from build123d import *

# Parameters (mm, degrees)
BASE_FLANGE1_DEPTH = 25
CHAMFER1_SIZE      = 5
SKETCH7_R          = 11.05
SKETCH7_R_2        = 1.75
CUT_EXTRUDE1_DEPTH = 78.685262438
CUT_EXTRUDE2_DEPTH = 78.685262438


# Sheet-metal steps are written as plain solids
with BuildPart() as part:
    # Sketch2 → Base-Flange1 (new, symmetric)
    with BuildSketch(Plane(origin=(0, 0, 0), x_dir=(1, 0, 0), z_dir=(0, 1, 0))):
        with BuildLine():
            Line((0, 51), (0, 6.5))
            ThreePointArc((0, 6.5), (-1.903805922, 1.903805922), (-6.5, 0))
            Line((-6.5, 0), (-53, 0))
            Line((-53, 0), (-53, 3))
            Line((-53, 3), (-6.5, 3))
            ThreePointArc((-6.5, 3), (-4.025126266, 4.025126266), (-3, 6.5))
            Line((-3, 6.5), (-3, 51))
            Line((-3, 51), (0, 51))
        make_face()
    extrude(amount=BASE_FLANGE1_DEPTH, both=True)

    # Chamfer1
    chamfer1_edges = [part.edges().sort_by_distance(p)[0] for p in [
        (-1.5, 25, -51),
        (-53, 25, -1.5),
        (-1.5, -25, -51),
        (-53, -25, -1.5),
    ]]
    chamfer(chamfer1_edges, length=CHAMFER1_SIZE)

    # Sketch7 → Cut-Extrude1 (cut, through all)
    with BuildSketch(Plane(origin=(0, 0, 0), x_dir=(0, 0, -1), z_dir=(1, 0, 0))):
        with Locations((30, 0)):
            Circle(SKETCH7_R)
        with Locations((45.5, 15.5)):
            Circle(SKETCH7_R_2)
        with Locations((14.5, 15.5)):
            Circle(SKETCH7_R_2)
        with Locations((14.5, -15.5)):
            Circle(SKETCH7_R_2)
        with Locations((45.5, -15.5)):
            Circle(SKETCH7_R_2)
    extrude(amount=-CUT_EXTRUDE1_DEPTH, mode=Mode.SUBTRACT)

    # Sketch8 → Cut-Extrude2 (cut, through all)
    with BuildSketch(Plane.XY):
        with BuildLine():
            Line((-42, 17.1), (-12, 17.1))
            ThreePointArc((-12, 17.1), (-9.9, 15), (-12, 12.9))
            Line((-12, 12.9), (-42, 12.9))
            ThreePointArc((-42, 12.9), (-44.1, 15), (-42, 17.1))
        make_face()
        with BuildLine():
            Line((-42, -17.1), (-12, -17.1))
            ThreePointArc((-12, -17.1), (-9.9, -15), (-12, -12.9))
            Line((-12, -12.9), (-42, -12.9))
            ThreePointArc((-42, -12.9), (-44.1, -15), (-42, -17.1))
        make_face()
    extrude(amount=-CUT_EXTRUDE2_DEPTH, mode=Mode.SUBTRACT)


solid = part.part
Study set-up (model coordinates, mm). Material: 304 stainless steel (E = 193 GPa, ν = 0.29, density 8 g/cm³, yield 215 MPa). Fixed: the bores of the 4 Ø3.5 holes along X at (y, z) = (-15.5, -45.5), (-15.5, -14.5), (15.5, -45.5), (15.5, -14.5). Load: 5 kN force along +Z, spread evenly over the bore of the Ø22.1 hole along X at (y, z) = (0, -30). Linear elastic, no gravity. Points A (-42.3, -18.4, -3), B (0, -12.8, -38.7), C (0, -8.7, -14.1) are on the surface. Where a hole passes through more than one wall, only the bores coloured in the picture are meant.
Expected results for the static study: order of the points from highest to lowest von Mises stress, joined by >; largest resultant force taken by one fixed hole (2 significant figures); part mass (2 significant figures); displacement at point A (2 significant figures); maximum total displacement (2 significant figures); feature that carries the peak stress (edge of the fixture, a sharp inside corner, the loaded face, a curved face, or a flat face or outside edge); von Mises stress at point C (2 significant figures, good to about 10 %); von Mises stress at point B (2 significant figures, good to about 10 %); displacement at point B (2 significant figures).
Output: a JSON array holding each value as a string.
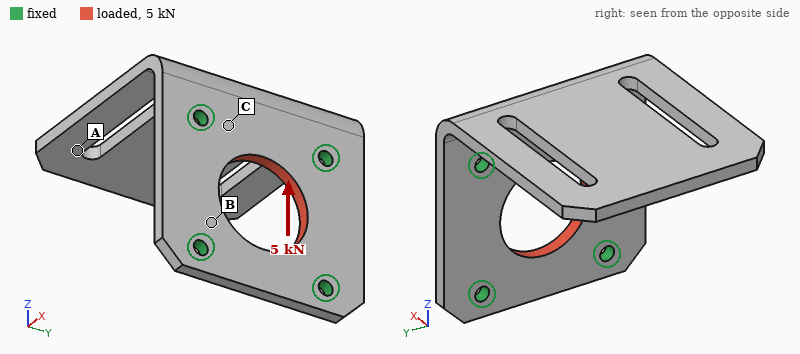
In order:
["B > C > A", "1.3 kN", "100 g", "1.8 µm", "5.4 µm", "edge of the fixture", "20 MPa", "36 MPa", "1.6 µm"]
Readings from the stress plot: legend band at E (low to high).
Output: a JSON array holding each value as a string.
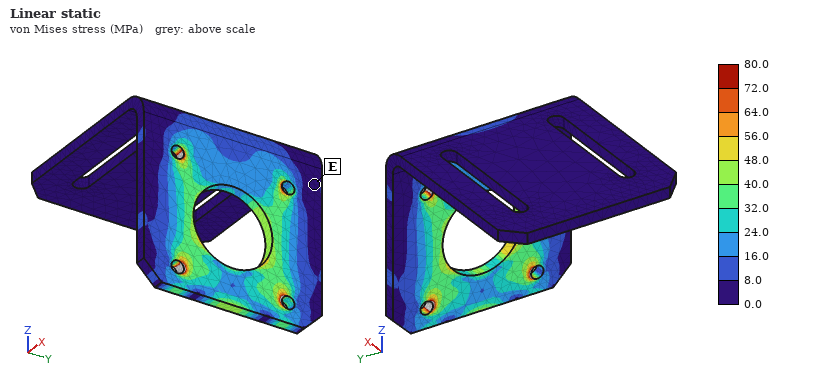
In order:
["0.0 to 8.0 MPa"]
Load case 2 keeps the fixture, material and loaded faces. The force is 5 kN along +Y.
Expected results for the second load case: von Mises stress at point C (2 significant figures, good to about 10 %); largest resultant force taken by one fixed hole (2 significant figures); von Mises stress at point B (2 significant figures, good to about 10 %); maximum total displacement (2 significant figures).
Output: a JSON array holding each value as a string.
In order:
["26 MPa", "1.3 kN", "27 MPa", "4.1 µm"]
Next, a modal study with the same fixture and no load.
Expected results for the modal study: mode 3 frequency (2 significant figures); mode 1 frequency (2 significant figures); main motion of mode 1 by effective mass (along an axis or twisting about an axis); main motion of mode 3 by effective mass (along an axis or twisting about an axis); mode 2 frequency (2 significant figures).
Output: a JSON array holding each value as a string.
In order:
["2600 Hz", "680 Hz", "along Z", "along Y", "1800 Hz"]
